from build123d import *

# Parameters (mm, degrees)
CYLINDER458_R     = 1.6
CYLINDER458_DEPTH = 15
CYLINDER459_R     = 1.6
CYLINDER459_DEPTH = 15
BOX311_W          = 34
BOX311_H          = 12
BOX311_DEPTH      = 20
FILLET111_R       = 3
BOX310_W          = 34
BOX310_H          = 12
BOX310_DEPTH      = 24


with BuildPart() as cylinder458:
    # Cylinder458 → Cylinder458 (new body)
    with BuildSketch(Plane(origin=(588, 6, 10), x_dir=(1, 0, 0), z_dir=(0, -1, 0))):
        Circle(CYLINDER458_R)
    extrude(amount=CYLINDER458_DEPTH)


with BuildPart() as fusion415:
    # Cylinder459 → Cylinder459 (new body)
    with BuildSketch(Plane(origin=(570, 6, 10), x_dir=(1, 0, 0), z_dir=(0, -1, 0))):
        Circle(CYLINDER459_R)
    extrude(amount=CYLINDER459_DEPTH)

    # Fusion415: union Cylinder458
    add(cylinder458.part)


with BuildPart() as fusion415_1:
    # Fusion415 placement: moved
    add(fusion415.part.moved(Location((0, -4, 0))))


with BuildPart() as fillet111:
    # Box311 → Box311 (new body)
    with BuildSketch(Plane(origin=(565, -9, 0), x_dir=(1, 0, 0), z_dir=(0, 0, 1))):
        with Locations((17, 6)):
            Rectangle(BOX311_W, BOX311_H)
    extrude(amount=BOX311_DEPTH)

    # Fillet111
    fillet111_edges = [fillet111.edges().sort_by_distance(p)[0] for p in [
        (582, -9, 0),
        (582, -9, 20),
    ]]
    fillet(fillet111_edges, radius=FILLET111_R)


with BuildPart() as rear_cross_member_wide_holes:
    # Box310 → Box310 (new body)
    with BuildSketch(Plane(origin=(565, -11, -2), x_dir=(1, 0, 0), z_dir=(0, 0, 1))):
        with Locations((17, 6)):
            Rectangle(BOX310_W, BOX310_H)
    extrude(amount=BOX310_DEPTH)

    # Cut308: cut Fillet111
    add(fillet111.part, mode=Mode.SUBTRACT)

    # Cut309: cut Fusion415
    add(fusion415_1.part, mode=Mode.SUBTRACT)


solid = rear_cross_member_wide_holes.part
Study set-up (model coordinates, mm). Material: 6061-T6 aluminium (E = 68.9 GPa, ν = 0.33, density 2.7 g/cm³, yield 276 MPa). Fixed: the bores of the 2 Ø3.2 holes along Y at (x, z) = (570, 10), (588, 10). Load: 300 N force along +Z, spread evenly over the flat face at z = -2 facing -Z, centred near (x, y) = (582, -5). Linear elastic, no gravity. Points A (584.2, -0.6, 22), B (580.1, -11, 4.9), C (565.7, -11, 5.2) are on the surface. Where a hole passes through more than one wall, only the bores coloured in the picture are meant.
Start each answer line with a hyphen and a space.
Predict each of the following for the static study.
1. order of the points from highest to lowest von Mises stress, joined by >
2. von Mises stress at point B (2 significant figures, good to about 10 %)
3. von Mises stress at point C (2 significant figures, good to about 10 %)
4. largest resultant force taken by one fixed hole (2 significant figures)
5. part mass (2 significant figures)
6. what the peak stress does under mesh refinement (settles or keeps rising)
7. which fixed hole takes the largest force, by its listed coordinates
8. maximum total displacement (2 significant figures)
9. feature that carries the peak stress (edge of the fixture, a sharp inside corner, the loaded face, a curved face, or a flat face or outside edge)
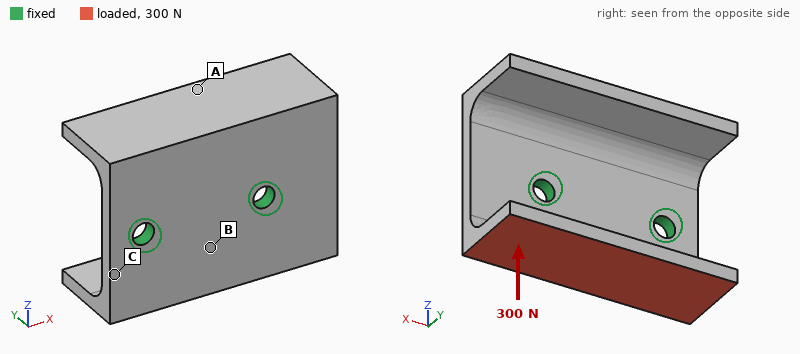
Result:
- C > B > A
- 53 MPa
- 67 MPa
- 200 N
- 8.3 g
- keeps rising
- (588, 10)
- 0.12 mm
- edge of the fixture
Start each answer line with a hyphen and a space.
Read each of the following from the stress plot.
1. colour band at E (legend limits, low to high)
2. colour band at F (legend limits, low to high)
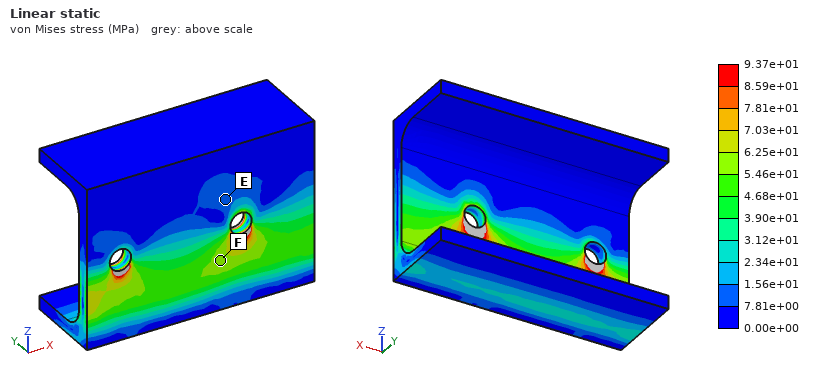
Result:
- 7.81e+00 to 1.56e+01 MPa
- 5.46e+01 to 6.25e+01 MPa
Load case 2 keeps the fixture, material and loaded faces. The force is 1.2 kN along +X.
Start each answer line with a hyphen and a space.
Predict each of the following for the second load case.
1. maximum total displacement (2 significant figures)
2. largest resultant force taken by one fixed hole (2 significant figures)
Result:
- 0.15 mm
- 1.0 kN
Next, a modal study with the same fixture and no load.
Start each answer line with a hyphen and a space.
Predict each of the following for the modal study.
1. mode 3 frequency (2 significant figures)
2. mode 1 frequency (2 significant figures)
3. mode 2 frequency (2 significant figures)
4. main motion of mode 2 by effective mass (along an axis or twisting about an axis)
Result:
- 7300 Hz
- 4400 Hz
- 5100 Hz
- along Y
